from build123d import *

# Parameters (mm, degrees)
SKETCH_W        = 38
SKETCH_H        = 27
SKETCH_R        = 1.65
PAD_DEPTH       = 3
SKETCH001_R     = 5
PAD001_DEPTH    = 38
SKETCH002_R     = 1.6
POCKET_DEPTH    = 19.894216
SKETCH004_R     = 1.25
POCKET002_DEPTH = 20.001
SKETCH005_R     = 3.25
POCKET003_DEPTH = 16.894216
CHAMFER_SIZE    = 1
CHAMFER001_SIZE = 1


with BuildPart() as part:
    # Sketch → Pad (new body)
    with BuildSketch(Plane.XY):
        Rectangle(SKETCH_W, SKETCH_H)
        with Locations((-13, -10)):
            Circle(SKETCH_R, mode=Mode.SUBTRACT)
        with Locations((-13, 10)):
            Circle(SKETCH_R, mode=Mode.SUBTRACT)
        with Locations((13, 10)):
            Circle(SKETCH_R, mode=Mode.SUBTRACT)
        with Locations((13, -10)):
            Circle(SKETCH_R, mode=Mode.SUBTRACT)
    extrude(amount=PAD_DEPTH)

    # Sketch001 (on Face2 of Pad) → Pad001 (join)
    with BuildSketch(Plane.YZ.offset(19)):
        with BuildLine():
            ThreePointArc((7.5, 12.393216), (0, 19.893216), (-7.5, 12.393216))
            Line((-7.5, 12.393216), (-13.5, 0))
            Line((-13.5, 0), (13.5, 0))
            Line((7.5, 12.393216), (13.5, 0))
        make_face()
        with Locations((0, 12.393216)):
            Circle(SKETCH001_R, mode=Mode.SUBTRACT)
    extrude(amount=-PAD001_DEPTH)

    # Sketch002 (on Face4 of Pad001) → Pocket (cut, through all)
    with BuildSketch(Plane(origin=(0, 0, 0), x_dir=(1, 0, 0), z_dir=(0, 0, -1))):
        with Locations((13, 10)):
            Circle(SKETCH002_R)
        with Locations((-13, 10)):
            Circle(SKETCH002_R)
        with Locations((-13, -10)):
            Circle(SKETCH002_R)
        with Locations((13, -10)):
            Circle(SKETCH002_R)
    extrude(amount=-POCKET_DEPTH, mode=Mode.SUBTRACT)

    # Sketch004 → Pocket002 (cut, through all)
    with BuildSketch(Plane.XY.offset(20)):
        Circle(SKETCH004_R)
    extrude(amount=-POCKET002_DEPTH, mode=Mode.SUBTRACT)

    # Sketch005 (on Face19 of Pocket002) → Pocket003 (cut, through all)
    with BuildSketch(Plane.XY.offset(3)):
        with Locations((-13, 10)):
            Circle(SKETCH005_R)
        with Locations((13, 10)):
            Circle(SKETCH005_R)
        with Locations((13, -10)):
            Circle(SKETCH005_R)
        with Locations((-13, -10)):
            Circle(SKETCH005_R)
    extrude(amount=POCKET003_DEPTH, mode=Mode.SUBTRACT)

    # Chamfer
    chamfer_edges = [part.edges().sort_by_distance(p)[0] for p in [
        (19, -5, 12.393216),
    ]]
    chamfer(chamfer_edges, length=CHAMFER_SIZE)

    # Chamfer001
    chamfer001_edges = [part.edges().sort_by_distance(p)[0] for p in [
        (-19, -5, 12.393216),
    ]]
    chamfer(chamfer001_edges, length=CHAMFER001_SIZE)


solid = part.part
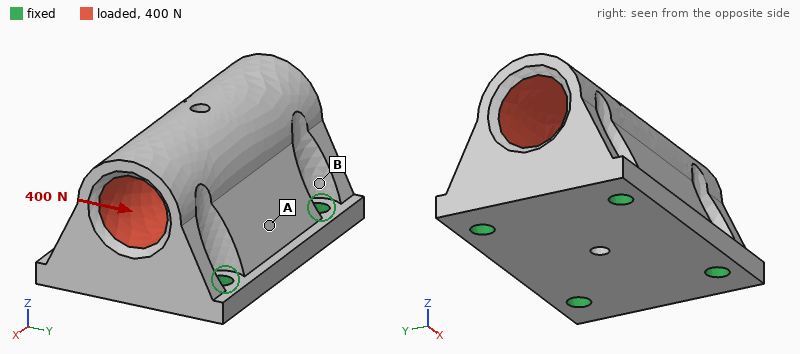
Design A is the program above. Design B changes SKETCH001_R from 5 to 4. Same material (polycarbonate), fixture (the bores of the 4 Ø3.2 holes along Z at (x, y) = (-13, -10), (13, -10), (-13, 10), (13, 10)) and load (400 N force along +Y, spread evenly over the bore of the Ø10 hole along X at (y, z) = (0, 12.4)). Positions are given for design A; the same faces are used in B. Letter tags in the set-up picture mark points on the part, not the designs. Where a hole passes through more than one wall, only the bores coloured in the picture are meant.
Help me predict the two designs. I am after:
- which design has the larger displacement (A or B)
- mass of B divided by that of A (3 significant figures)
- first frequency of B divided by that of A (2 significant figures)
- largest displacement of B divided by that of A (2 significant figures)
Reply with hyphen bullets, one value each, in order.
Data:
- A
- 1.11
- 1.0
- 0.77
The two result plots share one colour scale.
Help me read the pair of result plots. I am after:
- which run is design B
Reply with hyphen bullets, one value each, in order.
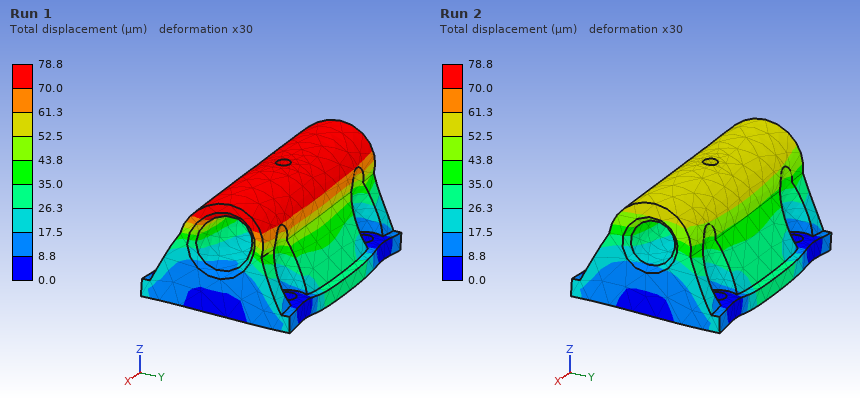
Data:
- Run 2
